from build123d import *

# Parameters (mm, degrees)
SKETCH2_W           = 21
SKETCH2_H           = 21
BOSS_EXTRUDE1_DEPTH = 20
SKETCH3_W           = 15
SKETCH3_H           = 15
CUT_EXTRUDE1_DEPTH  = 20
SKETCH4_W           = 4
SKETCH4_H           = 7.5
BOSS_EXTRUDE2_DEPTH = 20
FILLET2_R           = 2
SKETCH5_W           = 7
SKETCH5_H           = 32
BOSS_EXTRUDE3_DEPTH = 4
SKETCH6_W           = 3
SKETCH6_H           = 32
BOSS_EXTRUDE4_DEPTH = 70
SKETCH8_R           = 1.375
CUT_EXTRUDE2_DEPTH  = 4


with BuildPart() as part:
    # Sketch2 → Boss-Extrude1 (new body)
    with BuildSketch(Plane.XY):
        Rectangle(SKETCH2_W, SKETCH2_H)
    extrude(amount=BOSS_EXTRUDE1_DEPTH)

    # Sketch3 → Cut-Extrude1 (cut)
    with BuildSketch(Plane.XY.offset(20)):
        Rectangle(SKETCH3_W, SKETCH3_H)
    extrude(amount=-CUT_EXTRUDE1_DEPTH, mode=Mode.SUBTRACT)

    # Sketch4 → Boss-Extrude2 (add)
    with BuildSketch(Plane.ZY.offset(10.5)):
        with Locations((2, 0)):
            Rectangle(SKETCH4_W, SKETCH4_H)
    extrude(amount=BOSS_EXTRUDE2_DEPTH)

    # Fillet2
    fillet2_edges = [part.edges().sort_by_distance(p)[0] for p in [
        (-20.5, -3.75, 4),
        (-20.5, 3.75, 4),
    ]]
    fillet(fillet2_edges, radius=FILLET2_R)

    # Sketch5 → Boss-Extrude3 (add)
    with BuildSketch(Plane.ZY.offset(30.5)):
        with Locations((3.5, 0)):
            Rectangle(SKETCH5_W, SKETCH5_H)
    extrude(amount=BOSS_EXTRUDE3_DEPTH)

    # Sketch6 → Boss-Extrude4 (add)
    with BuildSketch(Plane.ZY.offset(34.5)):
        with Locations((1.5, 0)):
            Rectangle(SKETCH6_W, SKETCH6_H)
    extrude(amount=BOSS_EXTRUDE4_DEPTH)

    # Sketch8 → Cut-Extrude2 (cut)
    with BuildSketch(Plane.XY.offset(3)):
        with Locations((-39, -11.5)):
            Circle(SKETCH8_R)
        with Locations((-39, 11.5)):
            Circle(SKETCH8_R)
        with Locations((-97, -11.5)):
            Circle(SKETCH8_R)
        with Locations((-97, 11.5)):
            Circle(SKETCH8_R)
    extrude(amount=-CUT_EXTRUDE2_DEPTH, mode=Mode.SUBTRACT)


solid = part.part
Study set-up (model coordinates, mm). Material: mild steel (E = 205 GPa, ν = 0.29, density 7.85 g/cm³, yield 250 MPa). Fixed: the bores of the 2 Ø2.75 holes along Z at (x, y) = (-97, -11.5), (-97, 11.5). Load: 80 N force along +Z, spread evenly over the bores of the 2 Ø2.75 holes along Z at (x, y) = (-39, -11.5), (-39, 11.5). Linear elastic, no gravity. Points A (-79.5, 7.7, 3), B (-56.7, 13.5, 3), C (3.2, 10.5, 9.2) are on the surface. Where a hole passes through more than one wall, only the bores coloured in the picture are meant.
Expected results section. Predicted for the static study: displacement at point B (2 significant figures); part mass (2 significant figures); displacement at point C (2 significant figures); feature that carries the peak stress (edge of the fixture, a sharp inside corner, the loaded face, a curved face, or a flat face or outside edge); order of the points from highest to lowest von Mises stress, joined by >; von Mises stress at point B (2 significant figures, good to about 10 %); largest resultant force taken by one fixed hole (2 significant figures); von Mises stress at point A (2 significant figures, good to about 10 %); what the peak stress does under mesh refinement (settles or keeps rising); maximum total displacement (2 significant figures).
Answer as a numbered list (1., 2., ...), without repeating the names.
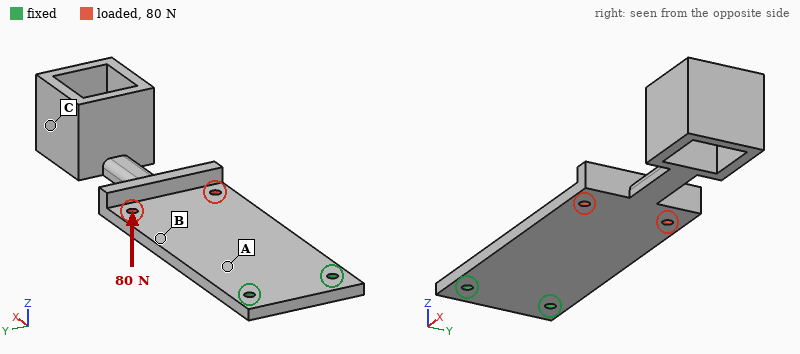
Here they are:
1. 0.21 mm
2. 98 g
3. 0.76 mm
4. edge of the fixture
5. A > B > C
6. 30 MPa
7. 40 N
8. 65 MPa
9. keeps rising
10. 0.84 mm
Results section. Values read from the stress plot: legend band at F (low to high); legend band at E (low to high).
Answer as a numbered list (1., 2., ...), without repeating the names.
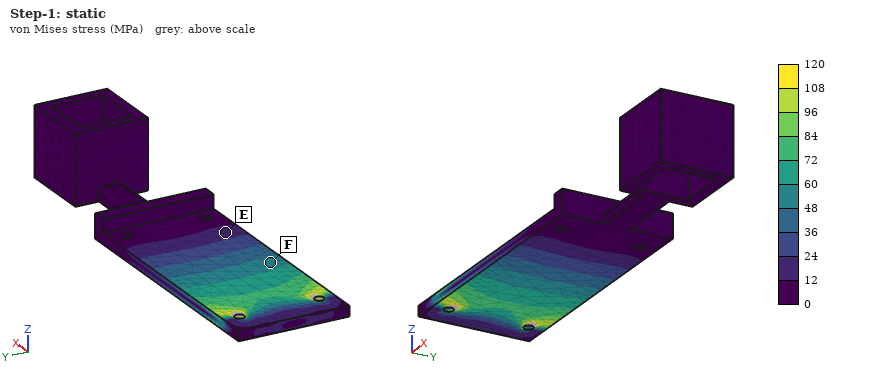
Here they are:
1. 48 to 60 MPa
2. 12 to 24 MPa
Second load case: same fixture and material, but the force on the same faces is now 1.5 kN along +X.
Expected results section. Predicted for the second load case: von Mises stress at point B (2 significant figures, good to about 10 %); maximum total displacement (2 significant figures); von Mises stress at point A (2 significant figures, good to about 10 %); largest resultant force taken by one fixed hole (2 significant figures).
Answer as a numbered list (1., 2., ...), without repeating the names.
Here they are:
1. 17 MPa
2. 5.5 µm
3. 15 MPa
4. 760 N
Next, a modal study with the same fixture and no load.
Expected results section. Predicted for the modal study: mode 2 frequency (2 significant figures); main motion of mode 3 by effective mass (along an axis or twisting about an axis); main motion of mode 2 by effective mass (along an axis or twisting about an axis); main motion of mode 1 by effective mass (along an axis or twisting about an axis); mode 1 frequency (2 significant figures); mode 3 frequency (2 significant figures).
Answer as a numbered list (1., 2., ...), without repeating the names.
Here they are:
1. 740 Hz
2. along Z
3. along Y
4. along Z
5. 170 Hz
6. 940 Hz
